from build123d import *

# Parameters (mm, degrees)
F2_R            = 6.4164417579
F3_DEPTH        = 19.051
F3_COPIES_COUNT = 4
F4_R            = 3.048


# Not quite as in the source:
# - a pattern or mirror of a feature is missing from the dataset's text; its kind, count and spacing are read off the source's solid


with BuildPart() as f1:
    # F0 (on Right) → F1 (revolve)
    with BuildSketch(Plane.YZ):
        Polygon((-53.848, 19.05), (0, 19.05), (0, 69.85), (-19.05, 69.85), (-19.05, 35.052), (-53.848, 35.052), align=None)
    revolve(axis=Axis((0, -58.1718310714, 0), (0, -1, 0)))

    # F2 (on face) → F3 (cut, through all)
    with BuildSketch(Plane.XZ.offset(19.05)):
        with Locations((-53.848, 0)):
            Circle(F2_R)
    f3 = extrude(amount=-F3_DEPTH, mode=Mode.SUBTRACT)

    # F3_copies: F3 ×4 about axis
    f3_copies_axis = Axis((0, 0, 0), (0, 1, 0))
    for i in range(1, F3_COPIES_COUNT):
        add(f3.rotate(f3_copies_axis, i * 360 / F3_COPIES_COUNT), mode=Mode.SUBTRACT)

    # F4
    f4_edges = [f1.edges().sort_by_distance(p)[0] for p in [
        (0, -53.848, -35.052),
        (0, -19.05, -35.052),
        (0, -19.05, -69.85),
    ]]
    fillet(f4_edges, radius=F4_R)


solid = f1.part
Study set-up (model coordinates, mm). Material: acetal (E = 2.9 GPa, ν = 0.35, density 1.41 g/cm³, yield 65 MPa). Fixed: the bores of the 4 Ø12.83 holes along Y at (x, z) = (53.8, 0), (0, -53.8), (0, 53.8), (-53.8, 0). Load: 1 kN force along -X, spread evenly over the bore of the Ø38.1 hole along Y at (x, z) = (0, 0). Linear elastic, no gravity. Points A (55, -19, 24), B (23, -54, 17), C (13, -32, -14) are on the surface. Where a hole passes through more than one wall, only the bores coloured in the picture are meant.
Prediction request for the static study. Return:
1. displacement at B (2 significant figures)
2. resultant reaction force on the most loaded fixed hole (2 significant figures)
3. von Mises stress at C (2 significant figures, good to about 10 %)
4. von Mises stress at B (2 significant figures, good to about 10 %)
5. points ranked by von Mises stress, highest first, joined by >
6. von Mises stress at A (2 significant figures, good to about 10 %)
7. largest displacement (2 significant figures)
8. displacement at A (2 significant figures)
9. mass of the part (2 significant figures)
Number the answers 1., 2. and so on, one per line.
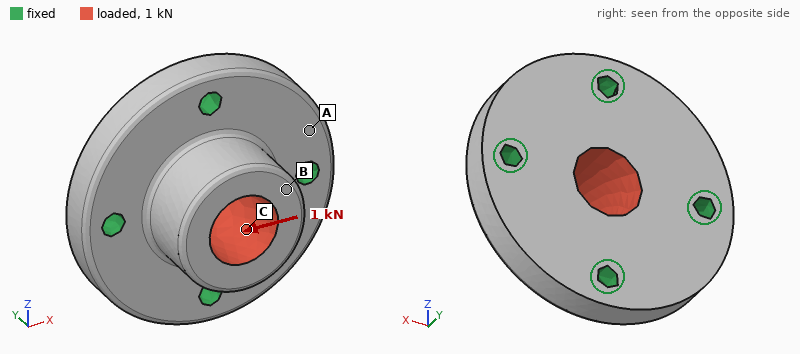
1. 19 µm
2. 360 N
3. 0.45 MPa
4. 0.27 MPa
5. C > B > A
6. 0.12 MPa
7. 20 µm
8. 3.1 µm
9. 500 g
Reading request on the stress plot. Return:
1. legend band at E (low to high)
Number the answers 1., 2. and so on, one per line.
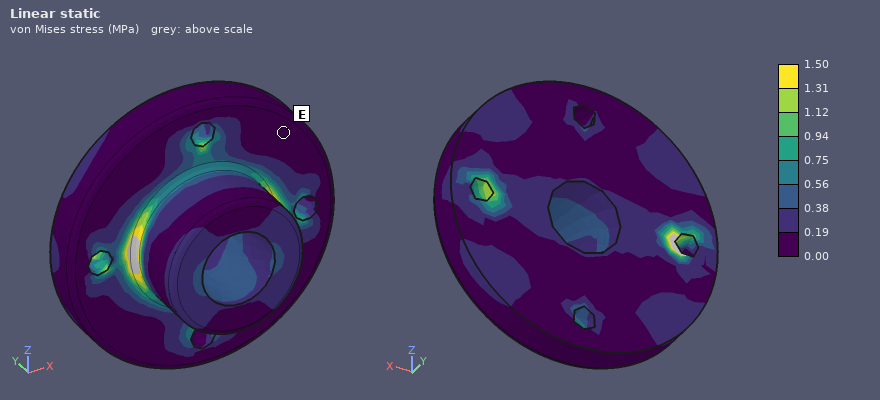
1. 0.00 to 0.19 MPa
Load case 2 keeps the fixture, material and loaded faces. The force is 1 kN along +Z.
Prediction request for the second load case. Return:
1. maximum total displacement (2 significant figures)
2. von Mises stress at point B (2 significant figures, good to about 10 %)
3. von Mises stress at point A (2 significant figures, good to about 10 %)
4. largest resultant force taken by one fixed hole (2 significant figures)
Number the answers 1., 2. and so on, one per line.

1. 20 µm
2. 0.20 MPa
3. 0.14 MPa
4. 360 N
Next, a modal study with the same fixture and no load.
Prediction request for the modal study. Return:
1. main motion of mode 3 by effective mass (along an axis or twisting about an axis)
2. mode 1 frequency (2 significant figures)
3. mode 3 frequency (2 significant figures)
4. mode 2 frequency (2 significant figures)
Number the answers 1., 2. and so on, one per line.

1. along Y
2. 2600 Hz
3. 2800 Hz
4. 2600 Hz
